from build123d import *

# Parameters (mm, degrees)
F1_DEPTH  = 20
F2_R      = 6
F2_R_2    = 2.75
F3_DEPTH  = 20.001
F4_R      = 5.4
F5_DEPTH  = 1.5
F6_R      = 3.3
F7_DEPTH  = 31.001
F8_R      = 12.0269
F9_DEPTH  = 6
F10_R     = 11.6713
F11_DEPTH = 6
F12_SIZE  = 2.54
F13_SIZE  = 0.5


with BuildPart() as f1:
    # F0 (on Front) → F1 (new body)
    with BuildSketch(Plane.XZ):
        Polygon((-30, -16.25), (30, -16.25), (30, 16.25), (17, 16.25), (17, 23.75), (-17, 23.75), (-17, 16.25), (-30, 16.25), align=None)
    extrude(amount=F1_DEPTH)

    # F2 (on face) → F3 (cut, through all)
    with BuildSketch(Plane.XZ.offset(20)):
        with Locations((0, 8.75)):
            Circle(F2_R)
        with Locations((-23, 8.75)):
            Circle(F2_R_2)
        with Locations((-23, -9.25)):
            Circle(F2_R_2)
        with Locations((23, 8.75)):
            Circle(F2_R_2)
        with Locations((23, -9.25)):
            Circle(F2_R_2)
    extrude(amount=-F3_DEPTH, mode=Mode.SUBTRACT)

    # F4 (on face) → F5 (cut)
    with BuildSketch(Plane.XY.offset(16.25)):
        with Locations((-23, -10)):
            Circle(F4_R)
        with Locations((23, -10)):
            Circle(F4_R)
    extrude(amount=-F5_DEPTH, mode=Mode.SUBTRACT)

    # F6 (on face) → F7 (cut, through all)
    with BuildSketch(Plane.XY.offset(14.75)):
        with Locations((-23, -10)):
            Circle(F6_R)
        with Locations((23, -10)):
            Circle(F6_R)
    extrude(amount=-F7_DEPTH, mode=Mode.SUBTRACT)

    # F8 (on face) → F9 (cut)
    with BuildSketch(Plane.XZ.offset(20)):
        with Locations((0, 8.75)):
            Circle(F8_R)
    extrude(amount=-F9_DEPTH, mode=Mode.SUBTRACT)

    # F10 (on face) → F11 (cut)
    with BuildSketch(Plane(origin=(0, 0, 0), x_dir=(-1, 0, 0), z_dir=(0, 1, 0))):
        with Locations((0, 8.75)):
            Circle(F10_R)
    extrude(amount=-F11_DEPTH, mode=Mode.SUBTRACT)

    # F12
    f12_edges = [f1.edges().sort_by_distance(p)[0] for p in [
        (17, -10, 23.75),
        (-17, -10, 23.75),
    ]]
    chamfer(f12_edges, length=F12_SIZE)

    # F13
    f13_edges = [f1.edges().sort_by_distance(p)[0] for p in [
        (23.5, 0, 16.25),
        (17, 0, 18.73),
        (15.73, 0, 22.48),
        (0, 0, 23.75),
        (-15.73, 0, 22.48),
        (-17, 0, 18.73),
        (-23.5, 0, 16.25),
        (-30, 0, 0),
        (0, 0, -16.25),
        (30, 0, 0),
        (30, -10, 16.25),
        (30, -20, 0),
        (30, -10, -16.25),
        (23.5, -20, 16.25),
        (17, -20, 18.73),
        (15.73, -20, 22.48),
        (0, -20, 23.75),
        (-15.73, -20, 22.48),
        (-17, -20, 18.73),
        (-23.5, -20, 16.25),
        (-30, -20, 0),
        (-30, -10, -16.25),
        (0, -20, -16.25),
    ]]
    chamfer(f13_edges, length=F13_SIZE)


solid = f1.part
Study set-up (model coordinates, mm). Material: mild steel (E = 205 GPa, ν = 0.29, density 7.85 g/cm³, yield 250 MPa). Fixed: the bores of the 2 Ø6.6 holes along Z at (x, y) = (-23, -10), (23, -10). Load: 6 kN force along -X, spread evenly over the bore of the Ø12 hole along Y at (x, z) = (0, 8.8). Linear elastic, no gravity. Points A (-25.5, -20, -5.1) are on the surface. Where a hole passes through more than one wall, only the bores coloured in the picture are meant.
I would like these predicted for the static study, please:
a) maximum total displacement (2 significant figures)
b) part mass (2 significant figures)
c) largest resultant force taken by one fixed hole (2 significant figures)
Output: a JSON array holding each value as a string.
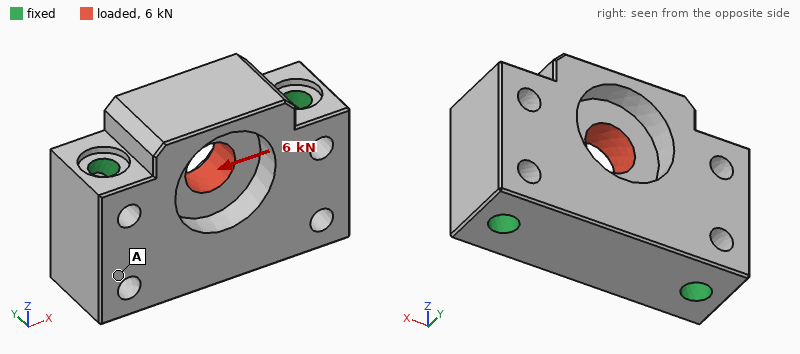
["1.9 µm", "270 g", "3.0 kN"]
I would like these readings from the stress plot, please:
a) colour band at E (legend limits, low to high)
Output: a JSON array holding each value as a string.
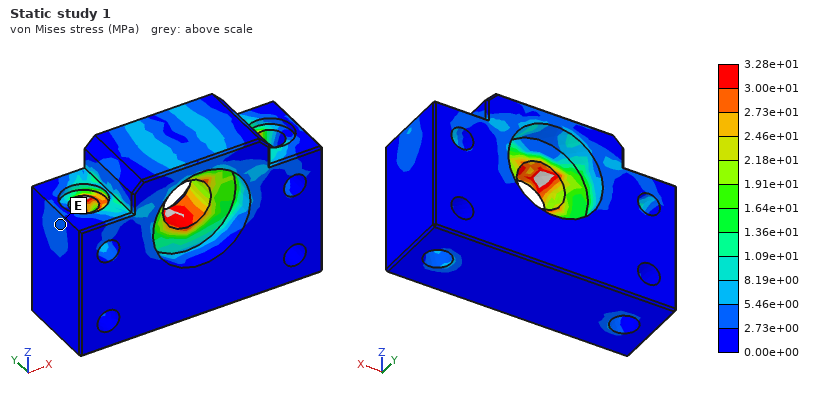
["2.73e+00 to 5.46e+00 MPa"]
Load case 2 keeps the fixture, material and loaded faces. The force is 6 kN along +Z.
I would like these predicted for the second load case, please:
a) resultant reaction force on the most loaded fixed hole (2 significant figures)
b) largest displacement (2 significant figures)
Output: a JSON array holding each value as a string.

["3.1 kN", "2.9 µm"]
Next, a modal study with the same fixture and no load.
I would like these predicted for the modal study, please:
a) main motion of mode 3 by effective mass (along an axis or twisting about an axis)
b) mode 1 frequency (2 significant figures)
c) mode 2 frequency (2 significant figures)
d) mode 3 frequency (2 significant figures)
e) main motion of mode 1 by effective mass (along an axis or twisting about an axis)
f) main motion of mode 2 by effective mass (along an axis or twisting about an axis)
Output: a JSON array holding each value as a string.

["along Z", "19 kHz", "26 kHz", "32 kHz", "along Y", "along Y"]
